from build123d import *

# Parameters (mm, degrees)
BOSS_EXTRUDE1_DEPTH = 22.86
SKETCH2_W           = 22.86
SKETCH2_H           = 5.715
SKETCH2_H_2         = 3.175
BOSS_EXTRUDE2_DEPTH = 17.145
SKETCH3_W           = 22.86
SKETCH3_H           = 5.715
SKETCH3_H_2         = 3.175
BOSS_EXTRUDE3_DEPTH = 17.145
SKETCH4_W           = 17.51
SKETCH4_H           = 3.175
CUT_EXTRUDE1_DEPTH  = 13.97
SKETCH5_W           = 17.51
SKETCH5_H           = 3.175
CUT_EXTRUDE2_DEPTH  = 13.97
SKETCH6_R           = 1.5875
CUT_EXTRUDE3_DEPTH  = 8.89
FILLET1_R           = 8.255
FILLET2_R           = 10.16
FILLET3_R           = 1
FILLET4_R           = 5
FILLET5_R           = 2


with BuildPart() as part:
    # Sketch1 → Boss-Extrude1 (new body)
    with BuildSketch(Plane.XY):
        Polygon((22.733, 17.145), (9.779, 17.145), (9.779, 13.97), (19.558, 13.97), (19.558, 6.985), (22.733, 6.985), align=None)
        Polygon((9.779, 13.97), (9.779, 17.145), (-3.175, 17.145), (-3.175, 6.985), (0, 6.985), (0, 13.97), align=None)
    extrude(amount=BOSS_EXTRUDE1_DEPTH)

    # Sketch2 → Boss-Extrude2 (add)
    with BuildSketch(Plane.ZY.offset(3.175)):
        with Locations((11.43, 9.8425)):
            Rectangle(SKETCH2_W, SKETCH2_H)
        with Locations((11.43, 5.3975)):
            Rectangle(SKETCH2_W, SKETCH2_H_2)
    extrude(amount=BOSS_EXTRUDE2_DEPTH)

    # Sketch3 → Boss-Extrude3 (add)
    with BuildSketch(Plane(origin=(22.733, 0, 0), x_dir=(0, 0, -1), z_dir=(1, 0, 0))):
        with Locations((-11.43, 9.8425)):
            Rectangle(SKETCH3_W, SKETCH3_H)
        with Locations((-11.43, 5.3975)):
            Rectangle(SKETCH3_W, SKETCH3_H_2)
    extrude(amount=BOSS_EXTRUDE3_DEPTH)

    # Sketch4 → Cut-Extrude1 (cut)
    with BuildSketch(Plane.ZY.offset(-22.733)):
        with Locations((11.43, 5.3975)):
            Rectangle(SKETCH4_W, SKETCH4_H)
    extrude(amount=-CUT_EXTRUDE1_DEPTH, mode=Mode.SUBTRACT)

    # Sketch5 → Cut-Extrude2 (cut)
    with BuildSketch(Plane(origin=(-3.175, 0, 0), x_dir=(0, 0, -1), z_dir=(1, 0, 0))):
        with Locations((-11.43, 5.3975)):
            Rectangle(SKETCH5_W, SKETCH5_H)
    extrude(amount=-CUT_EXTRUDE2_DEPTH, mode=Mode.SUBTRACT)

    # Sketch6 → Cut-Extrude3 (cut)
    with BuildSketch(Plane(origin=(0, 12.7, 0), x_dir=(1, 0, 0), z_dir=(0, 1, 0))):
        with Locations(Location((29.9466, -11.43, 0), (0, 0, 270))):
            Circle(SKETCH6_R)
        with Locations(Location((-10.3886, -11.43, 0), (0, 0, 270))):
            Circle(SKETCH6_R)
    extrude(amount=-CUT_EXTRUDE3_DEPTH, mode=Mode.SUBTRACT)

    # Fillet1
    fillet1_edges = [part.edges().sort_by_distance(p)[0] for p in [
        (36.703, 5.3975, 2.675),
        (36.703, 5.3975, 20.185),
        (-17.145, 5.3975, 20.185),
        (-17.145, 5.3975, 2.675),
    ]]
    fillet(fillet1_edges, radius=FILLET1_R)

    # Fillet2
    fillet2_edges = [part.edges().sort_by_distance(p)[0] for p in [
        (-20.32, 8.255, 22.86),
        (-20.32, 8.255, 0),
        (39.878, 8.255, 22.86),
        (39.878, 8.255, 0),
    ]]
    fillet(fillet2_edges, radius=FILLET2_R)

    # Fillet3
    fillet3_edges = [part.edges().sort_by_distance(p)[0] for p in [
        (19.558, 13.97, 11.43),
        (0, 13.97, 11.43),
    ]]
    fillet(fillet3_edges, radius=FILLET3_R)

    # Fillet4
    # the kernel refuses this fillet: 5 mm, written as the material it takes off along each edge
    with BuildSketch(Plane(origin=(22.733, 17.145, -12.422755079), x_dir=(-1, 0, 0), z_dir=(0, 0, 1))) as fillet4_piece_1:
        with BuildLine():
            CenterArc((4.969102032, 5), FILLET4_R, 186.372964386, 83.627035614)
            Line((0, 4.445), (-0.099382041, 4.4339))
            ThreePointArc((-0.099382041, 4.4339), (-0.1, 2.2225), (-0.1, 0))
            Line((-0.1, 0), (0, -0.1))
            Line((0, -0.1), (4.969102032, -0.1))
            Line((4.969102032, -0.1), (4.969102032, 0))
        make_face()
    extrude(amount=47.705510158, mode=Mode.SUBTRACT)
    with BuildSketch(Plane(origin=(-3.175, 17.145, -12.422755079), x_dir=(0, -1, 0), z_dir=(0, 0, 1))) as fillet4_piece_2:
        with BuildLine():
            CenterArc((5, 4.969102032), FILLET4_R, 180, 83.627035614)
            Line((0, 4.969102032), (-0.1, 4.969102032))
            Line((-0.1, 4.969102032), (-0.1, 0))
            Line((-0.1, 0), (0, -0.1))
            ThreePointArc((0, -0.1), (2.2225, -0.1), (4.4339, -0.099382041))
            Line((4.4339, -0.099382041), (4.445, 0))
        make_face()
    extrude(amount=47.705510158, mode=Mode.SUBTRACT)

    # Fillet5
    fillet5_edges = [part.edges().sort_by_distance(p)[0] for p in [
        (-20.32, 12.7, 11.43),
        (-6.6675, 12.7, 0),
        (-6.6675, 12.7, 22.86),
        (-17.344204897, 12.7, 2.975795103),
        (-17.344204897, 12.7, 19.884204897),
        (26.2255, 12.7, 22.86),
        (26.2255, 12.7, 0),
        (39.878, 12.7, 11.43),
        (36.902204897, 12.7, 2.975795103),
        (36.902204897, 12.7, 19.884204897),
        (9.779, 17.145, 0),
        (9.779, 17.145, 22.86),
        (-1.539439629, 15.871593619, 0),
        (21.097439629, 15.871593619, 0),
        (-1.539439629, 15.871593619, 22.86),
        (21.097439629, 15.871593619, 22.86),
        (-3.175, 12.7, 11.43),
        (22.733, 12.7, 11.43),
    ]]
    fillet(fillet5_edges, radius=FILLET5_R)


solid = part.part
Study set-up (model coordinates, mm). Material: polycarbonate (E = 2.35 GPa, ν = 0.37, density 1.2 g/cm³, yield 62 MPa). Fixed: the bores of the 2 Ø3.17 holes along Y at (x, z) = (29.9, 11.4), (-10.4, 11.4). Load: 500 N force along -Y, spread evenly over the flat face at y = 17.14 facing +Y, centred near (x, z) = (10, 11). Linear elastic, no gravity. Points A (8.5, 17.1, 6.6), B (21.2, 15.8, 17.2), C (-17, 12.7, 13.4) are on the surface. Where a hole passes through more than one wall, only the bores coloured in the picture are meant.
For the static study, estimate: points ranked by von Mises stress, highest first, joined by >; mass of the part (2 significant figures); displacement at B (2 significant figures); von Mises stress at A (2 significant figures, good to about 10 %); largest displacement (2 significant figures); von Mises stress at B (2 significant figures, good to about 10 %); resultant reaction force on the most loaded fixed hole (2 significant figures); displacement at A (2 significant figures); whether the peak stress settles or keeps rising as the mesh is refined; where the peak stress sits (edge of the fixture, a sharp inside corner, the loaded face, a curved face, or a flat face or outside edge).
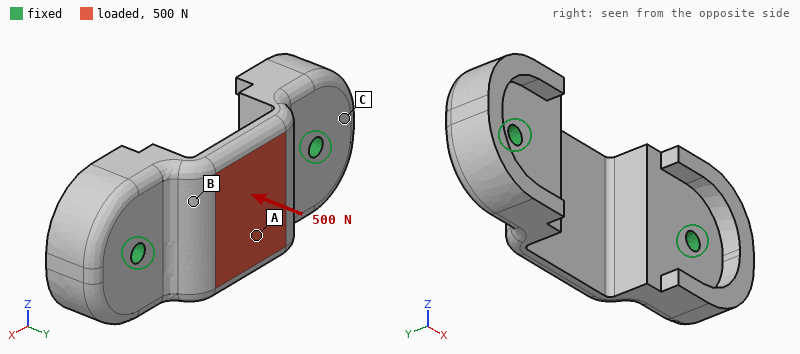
A > B > C
8.7 g
0.080 mm
21 MPa
0.28 mm
7.3 MPa
430 N
0.27 mm
keeps rising
edge of the fixture
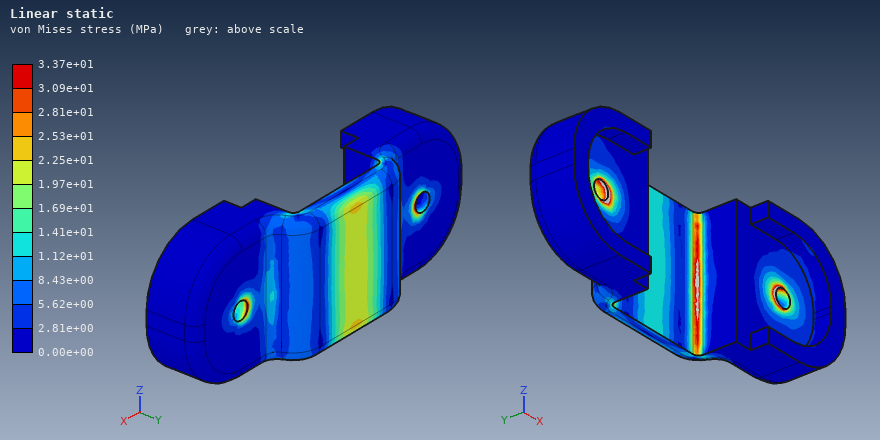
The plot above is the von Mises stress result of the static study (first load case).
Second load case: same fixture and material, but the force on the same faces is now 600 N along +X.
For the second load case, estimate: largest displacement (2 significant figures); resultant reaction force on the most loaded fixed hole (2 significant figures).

86 µm
310 N
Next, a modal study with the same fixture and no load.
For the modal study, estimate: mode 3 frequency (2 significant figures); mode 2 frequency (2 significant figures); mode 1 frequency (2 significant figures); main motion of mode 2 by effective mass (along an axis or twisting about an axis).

5500 Hz
5100 Hz
3500 Hz
along Y
